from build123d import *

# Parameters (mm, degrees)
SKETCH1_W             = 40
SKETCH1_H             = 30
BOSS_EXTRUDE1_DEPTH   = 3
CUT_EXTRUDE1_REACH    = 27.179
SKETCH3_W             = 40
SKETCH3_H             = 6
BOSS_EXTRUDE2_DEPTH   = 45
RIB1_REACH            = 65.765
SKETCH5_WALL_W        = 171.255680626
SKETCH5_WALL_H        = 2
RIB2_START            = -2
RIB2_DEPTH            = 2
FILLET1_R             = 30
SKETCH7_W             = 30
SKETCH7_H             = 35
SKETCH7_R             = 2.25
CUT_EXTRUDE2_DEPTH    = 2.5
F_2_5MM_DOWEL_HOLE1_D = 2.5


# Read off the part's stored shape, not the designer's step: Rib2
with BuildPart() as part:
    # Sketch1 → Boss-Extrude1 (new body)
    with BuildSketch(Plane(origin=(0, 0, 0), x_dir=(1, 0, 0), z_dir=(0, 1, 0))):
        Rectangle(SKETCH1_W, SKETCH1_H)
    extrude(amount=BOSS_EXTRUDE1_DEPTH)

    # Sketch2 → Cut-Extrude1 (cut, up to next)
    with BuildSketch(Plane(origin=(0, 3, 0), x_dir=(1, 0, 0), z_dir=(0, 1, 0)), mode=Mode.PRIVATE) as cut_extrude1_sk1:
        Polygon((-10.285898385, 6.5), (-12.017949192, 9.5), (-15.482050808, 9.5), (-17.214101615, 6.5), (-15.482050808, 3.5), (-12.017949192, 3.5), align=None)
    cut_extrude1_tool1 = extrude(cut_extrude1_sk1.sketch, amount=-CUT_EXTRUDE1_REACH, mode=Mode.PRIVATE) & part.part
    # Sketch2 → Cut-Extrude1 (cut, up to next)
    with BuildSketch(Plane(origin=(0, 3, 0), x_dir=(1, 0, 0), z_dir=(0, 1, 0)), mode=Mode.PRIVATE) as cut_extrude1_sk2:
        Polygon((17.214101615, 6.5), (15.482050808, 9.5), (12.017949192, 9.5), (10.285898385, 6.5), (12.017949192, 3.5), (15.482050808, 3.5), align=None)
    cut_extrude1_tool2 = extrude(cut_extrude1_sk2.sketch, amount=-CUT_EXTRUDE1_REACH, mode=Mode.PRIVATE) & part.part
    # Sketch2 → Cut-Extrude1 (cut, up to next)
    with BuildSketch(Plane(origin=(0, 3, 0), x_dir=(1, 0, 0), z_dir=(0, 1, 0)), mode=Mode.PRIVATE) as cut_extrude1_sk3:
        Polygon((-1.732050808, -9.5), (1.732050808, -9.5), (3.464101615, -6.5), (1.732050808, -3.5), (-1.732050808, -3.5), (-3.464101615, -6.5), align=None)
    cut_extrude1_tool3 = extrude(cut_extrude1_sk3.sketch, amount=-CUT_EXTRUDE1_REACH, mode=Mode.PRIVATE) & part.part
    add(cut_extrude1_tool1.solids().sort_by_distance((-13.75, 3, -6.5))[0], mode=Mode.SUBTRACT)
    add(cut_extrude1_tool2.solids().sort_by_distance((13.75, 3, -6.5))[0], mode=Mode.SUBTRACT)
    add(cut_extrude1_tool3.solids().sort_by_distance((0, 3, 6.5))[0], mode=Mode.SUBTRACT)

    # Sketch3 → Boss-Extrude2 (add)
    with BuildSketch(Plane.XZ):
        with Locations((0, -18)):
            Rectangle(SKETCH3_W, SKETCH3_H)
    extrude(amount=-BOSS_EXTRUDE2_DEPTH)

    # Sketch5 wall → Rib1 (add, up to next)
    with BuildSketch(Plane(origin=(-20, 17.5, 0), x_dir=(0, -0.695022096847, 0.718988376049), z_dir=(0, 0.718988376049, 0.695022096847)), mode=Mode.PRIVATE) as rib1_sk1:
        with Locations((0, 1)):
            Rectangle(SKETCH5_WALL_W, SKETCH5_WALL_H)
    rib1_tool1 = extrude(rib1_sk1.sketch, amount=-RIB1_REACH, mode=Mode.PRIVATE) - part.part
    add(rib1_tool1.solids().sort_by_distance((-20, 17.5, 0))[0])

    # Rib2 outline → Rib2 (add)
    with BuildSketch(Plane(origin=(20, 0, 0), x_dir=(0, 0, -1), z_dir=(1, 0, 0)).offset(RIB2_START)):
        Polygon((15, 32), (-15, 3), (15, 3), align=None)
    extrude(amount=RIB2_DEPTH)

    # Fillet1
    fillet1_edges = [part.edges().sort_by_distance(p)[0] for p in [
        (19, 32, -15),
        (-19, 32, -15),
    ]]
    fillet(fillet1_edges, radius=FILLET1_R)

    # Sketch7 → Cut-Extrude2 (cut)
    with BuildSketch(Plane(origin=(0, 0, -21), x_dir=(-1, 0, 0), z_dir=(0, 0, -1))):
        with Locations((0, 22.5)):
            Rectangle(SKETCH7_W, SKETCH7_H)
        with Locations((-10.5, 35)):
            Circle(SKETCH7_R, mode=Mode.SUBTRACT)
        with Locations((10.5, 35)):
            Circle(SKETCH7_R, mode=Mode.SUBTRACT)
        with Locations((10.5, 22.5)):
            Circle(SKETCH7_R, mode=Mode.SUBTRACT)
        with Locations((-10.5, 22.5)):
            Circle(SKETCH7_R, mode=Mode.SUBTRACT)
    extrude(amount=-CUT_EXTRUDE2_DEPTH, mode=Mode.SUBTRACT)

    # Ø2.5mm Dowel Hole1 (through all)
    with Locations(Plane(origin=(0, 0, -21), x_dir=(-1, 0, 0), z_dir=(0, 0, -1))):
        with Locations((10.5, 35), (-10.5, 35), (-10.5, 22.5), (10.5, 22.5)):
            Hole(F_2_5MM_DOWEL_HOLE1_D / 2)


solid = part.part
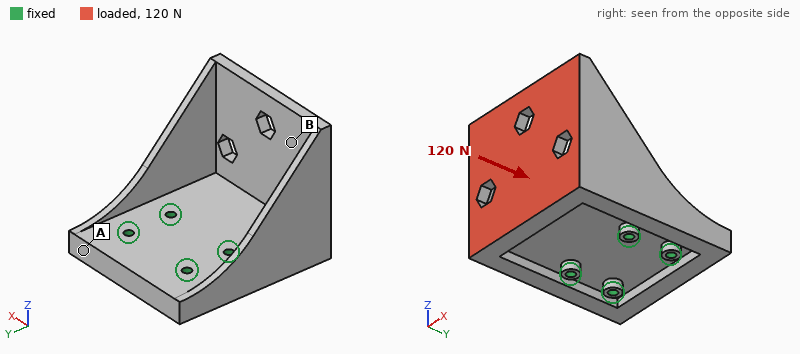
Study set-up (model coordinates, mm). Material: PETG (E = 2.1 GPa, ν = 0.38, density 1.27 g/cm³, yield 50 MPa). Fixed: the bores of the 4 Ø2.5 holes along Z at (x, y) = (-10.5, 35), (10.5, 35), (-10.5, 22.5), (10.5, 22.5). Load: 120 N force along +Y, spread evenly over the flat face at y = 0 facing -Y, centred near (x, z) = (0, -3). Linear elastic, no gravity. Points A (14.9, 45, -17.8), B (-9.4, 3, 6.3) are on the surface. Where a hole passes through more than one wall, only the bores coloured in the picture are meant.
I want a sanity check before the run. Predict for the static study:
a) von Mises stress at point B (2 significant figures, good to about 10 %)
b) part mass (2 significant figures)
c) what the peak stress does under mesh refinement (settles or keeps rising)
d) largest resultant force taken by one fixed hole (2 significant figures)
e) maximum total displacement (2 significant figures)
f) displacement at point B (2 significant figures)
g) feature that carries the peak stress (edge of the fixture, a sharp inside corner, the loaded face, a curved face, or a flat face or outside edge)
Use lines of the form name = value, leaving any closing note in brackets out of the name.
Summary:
von Mises stress at point B = 3.8 MPa
part mass = 17 g
what the peak stress does under mesh refinement = keeps rising
largest resultant force taken by one fixed hole = 60 N
maximum total displacement = 0.77 mm
displacement at point B = 0.49 mm
feature that carries the peak stress = edge of the fixture
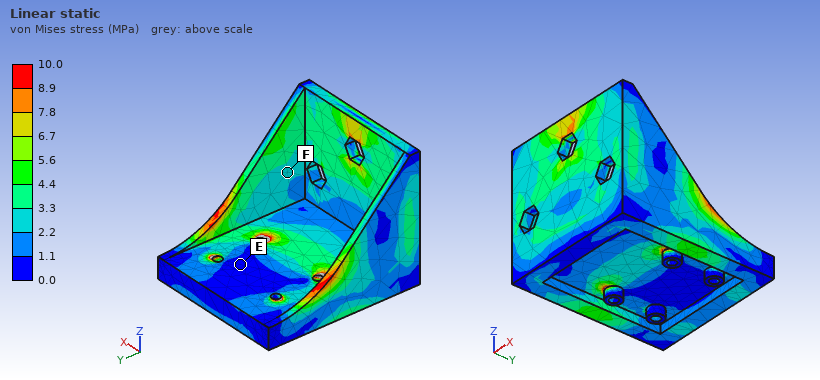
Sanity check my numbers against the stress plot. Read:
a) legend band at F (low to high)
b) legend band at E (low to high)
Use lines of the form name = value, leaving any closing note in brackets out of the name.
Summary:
legend band at F = 2.2 to 3.3 MPa
legend band at E = 0.0 to 1.1 MPa
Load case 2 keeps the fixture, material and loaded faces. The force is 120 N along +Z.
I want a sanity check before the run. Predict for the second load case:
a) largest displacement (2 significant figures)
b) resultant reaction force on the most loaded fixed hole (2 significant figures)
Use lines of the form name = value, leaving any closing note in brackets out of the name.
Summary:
largest displacement = 0.78 mm
resultant reaction force on the most loaded fixed hole = 130 N
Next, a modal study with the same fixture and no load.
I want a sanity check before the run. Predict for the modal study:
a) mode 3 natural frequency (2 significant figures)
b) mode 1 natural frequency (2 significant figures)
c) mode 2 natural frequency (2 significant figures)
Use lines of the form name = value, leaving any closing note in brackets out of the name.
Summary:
mode 3 natural frequency = 1800 Hz
mode 1 natural frequency = 820 Hz
mode 2 natural frequency = 820 Hz
